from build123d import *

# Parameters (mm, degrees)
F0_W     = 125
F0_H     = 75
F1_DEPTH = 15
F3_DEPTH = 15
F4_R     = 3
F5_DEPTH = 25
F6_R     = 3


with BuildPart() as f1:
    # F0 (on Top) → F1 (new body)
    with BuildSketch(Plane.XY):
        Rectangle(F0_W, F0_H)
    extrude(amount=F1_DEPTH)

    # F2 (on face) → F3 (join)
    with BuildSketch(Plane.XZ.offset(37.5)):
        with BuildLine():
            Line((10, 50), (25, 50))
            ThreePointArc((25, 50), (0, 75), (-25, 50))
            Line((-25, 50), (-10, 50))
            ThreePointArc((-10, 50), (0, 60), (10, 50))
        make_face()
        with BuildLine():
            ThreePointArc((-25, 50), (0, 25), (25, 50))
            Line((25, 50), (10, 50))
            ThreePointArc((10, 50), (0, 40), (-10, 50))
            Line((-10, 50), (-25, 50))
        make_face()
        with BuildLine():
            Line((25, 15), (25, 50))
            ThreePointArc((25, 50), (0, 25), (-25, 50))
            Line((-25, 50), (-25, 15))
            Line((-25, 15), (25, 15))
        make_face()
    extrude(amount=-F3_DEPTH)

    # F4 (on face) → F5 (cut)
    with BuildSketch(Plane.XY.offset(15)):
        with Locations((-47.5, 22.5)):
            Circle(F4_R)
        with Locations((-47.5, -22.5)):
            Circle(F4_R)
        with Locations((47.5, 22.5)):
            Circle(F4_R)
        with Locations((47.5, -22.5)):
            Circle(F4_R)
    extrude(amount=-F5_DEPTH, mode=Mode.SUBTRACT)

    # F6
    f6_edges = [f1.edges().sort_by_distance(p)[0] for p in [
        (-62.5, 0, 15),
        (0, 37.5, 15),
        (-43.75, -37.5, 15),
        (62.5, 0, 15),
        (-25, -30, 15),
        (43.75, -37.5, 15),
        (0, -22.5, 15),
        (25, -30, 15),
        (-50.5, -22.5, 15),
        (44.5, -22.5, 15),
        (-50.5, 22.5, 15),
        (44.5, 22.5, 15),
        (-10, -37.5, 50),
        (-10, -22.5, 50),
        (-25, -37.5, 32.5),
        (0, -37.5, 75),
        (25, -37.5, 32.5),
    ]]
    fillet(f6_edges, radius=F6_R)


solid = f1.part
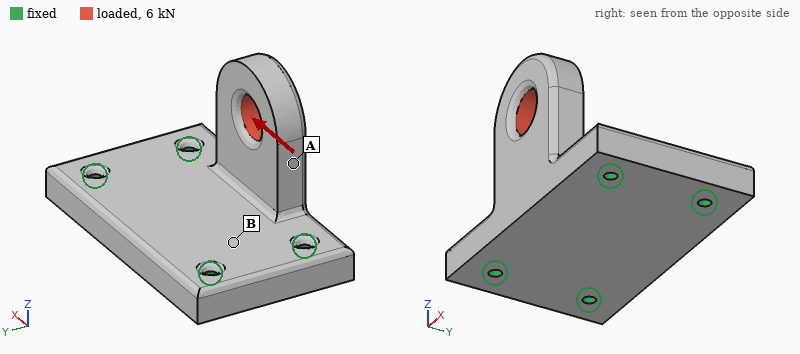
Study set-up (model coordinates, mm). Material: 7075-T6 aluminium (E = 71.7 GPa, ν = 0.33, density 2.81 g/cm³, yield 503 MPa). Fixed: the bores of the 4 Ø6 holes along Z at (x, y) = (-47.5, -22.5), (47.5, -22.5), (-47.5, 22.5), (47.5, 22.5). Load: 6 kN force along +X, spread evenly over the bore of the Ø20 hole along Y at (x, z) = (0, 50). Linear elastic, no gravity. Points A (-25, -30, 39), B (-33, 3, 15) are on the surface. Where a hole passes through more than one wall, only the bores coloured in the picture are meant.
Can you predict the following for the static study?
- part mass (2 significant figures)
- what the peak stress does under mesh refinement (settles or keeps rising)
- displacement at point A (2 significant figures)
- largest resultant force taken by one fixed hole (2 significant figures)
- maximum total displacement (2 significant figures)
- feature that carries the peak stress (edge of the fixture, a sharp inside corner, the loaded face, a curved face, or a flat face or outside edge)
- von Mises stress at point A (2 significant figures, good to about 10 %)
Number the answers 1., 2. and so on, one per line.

1. 490 g
2. keeps rising
3. 48 µm
4. 4.1 kN
5. 91 µm
6. a sharp inside corner
7. 20 MPa
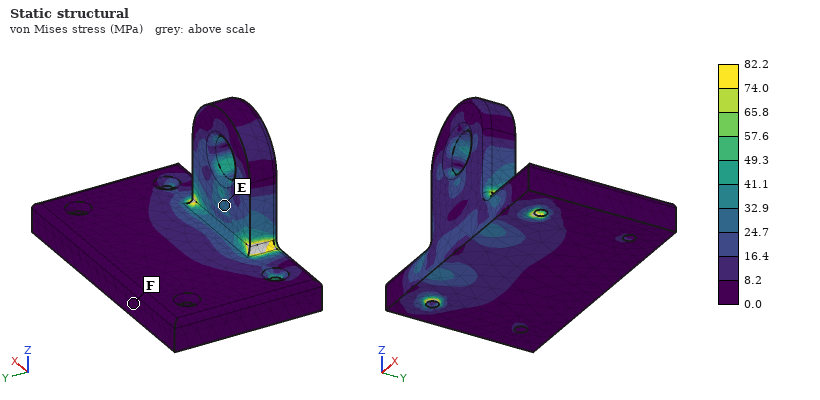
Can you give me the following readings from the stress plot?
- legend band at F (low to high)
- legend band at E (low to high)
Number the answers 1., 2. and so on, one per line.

1. 0.0 to 8.2 MPa
2. 24.7 to 32.9 MPa
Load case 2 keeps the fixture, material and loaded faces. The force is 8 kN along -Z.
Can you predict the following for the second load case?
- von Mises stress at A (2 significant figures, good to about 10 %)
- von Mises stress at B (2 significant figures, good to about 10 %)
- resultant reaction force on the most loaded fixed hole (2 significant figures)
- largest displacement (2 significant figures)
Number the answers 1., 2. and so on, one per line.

1. 8.3 MPa
2. 13 MPa
3. 4.6 kN
4. 93 µm
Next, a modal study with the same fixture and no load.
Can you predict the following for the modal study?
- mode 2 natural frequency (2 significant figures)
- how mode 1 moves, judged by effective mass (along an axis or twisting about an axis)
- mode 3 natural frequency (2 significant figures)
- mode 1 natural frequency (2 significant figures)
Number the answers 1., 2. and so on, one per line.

1. 5400 Hz
2. along Y
3. 5500 Hz
4. 2600 Hz
